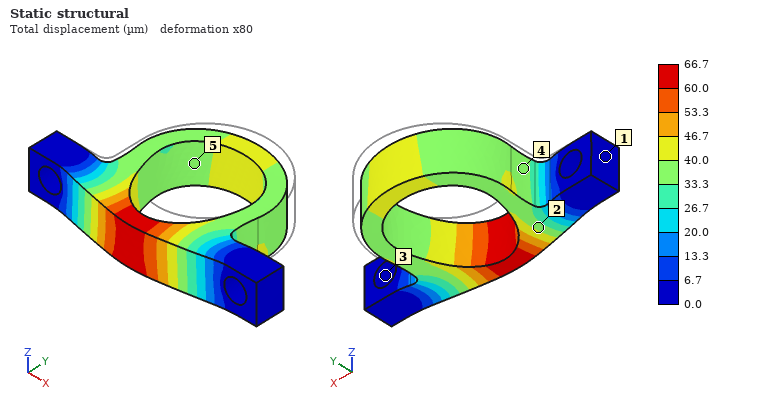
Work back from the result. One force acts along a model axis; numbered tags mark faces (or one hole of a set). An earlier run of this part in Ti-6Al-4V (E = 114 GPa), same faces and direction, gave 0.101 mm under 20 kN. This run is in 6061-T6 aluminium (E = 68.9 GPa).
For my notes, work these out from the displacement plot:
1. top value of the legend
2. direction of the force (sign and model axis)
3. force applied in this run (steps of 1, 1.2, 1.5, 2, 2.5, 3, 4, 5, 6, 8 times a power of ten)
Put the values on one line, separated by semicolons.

66.7 µm; -Y; 8 kN
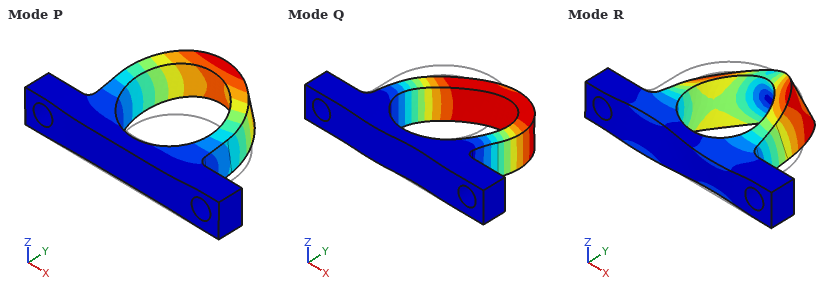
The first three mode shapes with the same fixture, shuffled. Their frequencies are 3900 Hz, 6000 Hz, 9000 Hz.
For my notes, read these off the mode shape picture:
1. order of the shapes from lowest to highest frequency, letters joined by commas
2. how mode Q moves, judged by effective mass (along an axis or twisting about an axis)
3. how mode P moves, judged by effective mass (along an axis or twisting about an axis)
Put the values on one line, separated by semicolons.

P, Q, R; along X; along Z
